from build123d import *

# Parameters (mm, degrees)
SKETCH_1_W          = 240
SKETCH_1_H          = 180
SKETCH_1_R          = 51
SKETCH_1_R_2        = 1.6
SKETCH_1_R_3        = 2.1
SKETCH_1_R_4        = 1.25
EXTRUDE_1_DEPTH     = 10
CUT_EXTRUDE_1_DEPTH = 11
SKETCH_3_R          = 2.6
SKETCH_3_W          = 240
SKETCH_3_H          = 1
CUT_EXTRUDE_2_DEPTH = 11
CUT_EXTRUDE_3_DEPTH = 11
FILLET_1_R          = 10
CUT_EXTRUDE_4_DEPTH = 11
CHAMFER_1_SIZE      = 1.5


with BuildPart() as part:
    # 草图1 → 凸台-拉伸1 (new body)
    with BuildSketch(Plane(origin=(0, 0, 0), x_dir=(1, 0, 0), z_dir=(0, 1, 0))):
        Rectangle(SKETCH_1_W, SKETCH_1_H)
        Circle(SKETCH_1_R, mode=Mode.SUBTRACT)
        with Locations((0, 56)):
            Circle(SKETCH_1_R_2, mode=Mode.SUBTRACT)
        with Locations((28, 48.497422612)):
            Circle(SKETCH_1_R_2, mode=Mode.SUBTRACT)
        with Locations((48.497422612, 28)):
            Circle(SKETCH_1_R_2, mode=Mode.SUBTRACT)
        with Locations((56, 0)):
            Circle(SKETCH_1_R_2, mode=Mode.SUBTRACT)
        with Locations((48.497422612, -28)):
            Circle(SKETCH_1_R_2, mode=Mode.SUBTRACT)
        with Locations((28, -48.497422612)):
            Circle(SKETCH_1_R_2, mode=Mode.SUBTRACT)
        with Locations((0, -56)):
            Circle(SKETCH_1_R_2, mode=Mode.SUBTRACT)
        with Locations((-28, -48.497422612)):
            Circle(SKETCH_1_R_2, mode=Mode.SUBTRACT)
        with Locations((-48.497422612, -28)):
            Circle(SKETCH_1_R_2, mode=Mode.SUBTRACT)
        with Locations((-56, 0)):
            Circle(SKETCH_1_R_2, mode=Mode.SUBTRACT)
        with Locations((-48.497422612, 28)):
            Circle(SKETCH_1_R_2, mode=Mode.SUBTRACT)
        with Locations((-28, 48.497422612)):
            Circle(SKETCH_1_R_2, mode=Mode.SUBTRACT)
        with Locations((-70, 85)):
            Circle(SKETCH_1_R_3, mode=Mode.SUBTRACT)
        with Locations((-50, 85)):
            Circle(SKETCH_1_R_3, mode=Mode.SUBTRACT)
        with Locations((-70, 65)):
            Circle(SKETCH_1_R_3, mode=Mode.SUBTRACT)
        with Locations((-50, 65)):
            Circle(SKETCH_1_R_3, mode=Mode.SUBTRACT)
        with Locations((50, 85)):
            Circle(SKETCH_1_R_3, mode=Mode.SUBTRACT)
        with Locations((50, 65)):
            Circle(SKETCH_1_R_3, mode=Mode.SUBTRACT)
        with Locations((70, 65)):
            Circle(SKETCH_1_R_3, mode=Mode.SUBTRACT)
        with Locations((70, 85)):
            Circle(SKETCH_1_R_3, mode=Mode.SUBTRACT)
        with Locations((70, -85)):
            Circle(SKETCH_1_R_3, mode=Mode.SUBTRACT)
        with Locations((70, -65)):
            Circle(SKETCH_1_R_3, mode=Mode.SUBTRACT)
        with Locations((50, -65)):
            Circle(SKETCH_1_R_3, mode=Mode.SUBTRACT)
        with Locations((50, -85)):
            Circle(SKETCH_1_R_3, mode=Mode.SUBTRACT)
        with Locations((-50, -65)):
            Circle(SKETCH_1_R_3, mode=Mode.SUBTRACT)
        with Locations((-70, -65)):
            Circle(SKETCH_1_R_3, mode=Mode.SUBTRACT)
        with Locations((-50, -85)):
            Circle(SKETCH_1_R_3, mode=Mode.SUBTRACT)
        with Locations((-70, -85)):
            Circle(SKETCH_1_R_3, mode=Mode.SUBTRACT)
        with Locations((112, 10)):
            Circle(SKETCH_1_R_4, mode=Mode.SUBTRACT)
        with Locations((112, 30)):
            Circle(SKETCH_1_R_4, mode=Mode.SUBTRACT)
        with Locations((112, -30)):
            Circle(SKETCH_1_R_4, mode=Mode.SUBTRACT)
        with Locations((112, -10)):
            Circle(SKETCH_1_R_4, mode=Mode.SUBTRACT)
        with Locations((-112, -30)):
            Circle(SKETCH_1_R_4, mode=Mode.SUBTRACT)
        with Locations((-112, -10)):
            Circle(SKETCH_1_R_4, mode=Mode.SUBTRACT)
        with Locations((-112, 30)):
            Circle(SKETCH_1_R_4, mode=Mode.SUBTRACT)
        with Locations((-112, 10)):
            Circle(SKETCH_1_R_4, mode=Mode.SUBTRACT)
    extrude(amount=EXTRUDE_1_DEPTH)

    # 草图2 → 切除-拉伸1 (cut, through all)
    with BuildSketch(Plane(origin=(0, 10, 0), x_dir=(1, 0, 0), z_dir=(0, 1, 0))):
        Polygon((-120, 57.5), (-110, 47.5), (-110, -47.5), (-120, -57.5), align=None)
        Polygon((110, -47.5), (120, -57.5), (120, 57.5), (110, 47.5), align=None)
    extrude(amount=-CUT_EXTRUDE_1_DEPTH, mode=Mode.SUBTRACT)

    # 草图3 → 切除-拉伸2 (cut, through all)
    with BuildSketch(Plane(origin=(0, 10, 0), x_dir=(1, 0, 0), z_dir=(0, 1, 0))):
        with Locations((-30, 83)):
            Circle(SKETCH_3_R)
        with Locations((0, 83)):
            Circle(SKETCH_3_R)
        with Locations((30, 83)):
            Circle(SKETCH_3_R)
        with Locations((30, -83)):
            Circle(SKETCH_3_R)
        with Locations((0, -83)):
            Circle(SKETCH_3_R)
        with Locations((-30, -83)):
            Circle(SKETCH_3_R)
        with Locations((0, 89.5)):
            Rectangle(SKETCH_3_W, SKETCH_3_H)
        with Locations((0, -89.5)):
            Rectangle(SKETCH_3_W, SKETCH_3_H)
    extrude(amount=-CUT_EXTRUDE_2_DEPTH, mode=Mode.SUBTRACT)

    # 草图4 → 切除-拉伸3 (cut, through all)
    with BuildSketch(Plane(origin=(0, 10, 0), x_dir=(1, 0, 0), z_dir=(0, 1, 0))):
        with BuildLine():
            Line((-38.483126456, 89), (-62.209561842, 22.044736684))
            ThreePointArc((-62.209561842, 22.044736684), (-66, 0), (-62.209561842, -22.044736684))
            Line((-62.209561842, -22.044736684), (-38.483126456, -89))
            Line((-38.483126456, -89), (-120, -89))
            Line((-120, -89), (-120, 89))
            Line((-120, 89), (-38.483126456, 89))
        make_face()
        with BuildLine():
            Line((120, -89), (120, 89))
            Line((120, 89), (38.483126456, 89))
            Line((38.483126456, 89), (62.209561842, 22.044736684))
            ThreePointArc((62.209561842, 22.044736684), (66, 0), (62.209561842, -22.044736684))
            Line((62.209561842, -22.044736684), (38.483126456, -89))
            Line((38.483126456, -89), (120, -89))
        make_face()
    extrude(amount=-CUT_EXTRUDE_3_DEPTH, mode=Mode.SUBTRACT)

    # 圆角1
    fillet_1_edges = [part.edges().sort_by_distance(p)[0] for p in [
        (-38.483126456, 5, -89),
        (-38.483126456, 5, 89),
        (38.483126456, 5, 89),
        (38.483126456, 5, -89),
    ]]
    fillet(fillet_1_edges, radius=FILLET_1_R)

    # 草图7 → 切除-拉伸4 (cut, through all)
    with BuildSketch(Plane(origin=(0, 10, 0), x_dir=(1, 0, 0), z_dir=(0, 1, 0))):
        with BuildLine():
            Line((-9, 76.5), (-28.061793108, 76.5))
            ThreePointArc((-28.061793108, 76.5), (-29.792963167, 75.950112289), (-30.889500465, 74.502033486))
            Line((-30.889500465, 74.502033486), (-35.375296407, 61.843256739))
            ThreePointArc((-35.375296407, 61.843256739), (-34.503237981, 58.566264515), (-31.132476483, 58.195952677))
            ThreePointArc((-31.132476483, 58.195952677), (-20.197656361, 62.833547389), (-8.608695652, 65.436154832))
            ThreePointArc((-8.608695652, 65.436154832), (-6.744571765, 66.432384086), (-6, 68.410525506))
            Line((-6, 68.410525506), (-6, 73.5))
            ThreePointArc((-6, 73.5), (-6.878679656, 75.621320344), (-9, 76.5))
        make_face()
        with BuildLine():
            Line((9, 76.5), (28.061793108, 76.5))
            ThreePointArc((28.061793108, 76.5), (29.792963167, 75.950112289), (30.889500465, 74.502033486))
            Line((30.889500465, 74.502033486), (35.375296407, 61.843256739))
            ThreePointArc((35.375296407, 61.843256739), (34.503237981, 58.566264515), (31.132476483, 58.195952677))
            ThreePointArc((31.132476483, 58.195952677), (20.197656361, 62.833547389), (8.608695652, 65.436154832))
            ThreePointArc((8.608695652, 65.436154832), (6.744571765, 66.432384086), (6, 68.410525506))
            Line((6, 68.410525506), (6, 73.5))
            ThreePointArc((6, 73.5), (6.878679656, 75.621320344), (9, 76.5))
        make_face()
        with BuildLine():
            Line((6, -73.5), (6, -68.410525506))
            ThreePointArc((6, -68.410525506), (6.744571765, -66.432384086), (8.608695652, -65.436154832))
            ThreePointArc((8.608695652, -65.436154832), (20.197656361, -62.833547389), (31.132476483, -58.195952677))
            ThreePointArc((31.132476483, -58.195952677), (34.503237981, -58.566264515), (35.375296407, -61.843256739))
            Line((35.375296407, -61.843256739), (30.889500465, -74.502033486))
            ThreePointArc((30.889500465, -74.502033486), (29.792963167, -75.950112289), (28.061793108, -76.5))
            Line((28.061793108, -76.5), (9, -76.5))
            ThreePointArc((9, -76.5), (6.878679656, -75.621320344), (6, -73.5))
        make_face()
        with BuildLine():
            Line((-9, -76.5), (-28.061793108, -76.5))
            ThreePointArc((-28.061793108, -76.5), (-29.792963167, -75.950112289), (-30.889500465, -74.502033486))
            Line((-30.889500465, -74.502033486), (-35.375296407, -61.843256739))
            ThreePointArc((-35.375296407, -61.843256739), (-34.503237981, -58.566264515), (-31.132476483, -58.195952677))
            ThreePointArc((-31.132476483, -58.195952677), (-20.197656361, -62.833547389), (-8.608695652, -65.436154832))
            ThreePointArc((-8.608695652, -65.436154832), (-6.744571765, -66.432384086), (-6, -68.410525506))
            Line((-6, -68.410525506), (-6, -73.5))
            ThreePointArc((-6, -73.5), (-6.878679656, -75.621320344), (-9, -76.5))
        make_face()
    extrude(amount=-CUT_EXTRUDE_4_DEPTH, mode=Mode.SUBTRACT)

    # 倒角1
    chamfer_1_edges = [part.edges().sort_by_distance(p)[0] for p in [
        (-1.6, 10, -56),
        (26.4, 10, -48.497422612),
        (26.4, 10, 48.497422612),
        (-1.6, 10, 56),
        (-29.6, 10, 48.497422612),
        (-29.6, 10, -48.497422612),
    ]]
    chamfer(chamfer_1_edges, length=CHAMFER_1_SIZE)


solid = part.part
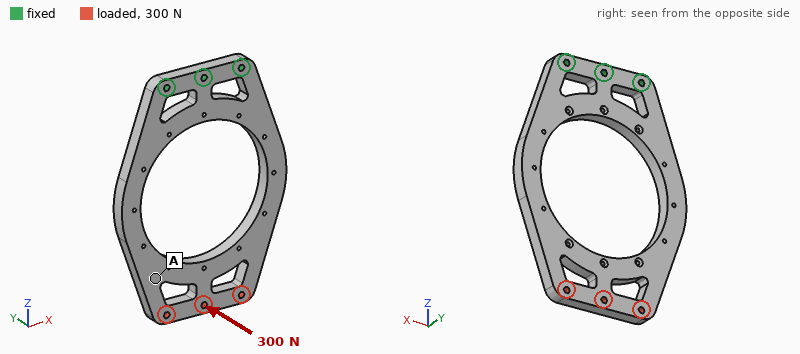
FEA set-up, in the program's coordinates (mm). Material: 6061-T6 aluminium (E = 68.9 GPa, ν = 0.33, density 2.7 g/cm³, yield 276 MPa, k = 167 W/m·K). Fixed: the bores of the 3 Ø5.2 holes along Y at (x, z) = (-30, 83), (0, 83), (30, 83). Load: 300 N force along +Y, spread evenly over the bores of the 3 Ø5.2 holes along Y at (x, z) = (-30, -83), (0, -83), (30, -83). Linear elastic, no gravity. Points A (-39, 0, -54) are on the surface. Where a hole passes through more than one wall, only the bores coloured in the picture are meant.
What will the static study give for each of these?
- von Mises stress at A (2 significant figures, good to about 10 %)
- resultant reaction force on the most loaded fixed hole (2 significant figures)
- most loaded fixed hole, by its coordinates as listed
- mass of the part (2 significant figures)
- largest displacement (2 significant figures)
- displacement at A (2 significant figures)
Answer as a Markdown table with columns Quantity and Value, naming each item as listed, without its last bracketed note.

| Quantity | Value |
|---|---|
| von Mises stress at A | 14 MPa |
| resultant reaction force on the most loaded fixed hole | 380 N |
| most loaded fixed hole, by its coordinates as listed | (0, 83) |
| mass of the part | 250 g |
| largest displacement | 2.6 mm |
| displacement at A | 1.8 mm |
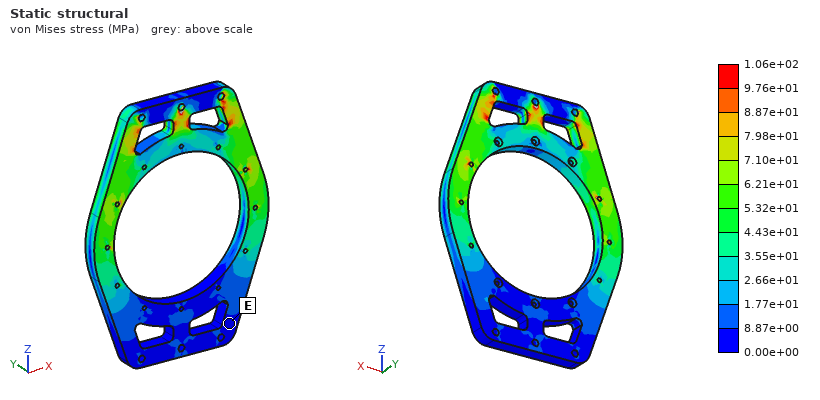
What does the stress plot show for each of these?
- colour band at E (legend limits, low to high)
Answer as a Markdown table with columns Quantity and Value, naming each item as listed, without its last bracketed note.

| Quantity | Value |
|---|---|
| colour band at E | 0.00e+00 to 8.87e+00 MPa |
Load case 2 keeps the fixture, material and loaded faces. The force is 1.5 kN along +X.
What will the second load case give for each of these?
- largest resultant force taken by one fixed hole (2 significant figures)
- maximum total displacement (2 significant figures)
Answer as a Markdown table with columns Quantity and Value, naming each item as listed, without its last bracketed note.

| Quantity | Value |
|---|---|
| largest resultant force taken by one fixed hole | 3.6 kN |
| maximum total displacement | 0.48 mm |
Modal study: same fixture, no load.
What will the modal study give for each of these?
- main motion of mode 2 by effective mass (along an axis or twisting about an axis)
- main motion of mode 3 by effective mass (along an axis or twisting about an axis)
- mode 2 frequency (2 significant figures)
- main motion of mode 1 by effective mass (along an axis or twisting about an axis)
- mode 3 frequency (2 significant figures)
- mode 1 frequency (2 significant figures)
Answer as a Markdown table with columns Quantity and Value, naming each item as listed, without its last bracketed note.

| Quantity | Value |
|---|---|
| main motion of mode 2 by effective mass | twisting about Z |
| main motion of mode 3 by effective mass | along X |
| mode 2 frequency | 660 Hz |
| main motion of mode 1 by effective mass | along Y |
| mode 3 frequency | 870 Hz |
| mode 1 frequency | 210 Hz |
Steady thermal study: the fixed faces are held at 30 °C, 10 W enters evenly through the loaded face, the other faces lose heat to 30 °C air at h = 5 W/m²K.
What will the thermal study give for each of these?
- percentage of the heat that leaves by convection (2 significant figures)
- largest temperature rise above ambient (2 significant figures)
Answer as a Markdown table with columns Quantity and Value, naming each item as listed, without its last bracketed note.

| Quantity | Value |
|---|---|
| percentage of the heat that leaves by convection | 20 % |
| largest temperature rise above ambient | 26 K |
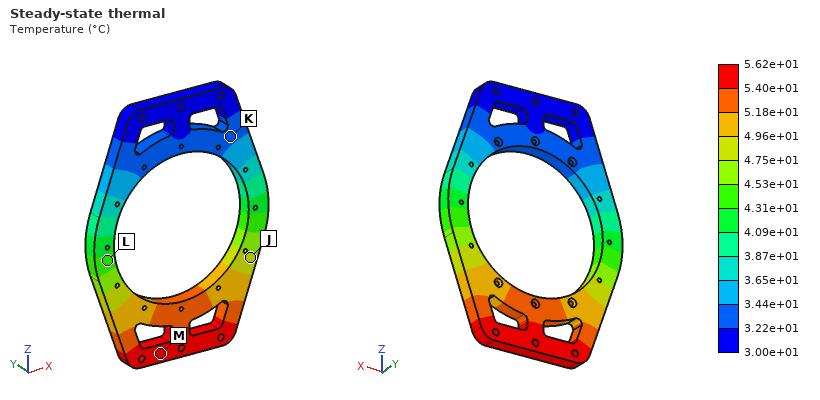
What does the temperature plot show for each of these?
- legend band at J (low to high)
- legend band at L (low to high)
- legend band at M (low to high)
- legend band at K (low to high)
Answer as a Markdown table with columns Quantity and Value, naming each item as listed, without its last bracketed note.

| Quantity | Value |
|---|---|
| legend band at J | 4.75e+01 to 4.96e+01 °C |
| legend band at L | 4.31e+01 to 4.53e+01 °C |
| legend band at M | 5.40e+01 to 5.62e+01 °C |
| legend band at K | 3.22e+01 to 3.44e+01 °C |
